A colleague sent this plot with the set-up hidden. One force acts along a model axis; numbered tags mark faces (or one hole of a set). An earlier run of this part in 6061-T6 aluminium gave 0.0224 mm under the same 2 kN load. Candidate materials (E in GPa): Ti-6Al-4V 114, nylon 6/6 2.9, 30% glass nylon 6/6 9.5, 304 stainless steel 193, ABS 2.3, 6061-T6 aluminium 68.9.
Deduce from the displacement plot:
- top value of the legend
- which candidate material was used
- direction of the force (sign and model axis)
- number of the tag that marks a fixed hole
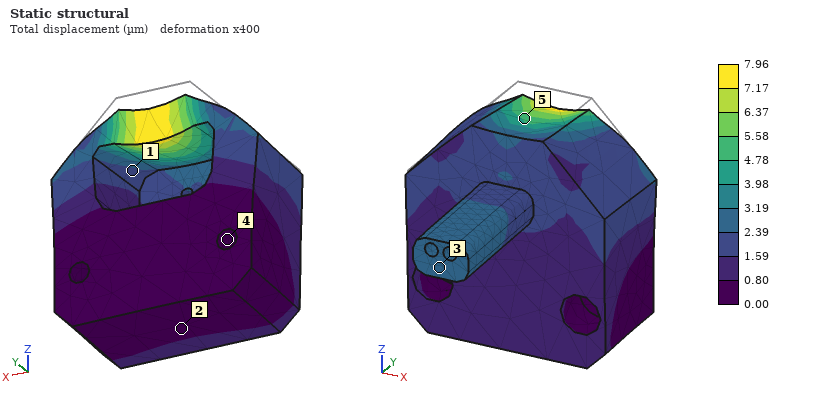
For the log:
7.96 µm
304 stainless steel
-Z
4
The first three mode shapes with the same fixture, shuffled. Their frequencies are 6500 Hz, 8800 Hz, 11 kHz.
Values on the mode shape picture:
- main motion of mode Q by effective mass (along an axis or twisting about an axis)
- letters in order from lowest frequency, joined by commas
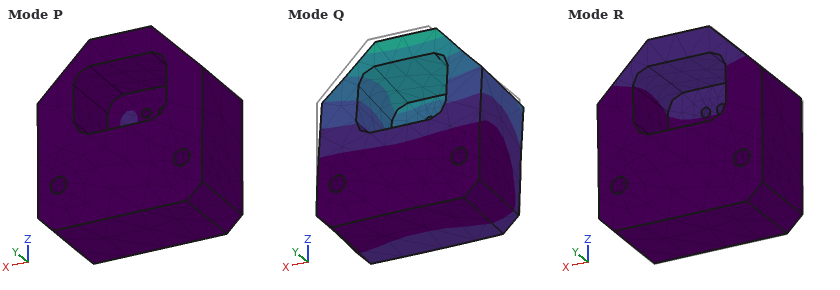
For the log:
along Y
R, P, Q
